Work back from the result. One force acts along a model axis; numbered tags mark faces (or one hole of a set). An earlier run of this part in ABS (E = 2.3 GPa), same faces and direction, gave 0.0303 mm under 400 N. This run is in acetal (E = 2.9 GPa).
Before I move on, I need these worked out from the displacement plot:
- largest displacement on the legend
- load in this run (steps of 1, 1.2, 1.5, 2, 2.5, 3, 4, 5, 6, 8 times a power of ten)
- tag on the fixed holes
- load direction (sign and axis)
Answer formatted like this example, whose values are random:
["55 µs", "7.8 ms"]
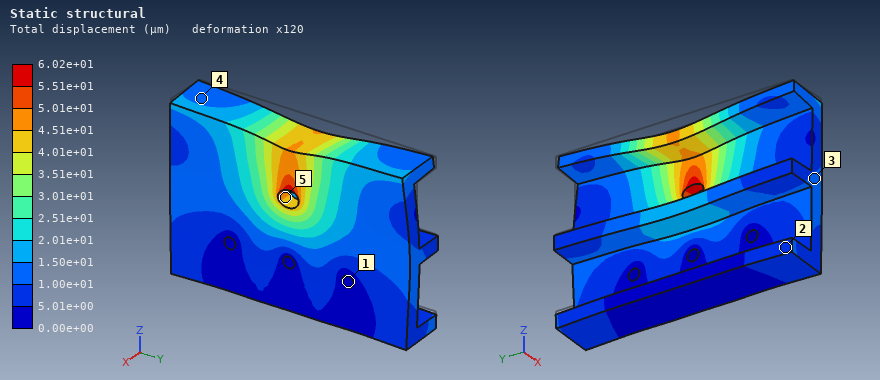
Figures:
["6.02e+01 µm", "1 kN", "1", "-Z"]
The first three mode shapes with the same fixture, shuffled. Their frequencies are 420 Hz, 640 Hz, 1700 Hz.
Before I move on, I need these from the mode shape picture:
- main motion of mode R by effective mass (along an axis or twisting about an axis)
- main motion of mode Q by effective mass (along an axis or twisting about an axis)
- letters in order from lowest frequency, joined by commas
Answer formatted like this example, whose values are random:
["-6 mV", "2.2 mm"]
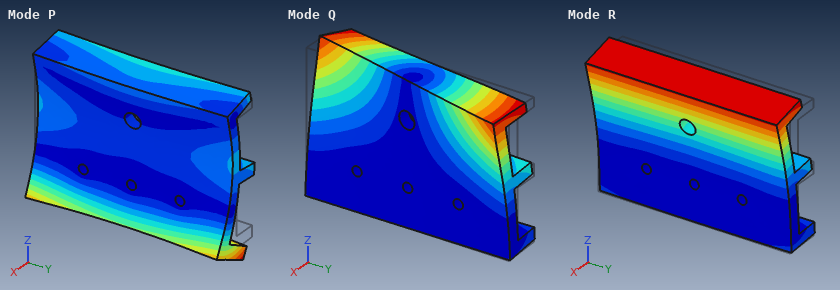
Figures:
["along X", "twisting about Z", "R, Q, P"]
